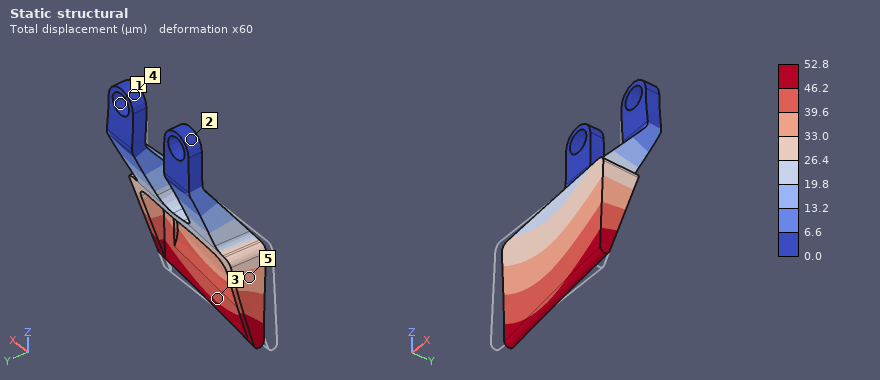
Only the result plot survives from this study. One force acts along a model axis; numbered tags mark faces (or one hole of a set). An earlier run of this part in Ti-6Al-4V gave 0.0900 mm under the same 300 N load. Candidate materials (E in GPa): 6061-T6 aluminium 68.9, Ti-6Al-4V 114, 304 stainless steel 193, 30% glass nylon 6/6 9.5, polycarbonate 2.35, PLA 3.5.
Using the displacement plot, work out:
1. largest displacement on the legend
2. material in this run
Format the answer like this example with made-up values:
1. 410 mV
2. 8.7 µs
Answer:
1. 52.8 µm
2. 304 stainless steel
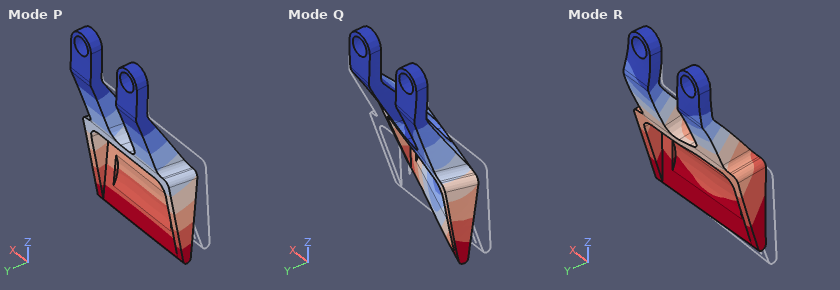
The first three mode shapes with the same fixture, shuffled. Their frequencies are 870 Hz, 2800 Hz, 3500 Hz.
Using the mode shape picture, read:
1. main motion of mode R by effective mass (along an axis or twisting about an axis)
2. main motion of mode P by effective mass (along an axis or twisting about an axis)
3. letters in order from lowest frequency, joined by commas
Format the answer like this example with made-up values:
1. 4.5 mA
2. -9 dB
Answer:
1. along X
2. along Y
3. P, Q, R
